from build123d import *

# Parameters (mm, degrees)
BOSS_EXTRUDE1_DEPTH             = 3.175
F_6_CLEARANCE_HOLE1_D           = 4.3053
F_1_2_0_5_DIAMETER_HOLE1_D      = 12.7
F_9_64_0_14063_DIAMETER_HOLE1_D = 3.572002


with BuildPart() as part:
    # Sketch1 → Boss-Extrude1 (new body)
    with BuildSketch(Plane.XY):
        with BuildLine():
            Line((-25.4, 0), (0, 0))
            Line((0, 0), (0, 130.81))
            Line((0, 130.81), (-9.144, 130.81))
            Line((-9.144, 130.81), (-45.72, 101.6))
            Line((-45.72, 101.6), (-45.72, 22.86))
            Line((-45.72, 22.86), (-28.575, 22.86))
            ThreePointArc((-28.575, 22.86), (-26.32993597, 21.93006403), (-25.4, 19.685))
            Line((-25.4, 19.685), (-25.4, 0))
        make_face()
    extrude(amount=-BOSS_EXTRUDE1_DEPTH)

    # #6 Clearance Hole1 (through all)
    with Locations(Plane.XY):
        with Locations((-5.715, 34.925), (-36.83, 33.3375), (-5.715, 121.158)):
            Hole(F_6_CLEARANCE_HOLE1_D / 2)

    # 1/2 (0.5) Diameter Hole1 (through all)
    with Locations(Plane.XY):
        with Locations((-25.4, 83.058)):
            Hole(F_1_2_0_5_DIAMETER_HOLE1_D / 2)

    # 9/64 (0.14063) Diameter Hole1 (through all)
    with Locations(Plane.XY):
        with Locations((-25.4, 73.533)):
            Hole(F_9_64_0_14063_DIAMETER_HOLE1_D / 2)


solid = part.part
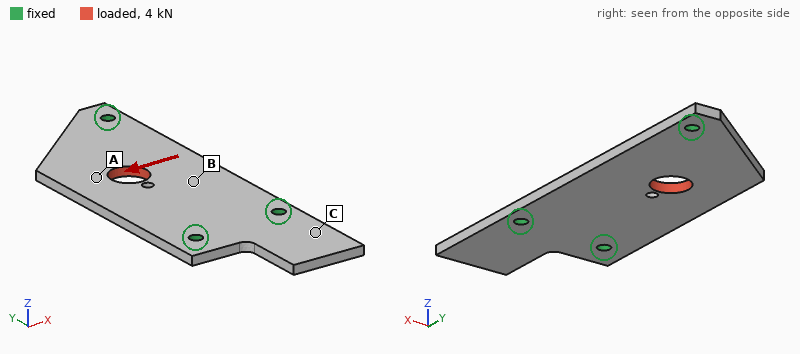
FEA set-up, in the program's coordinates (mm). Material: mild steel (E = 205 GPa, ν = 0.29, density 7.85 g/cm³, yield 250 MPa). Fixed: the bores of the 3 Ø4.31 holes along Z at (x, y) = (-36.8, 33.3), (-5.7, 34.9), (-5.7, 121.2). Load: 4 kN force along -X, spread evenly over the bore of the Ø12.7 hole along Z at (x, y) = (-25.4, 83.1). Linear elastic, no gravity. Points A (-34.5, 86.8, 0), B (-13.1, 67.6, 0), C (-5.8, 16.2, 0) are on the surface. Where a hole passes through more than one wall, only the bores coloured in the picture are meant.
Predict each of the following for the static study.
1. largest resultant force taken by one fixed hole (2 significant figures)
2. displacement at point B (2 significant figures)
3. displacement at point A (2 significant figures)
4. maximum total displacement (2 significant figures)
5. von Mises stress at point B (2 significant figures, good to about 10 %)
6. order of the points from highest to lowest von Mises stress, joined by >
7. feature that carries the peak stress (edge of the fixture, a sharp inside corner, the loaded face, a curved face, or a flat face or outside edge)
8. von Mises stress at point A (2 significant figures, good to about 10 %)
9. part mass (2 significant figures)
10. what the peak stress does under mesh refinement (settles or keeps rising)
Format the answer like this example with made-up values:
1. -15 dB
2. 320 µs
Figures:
1. 2.2 kN
2. 11 µm
3. 14 µm
4. 15 µm
5. 30 MPa
6. A > B > C
7. edge of the fixture
8. 43 MPa
9. 120 g
10. keeps rising
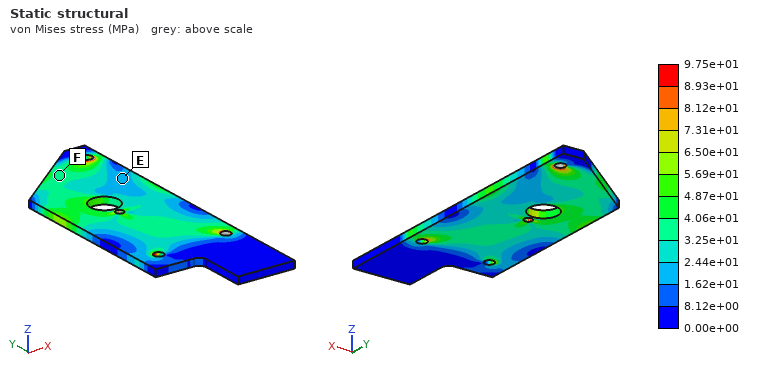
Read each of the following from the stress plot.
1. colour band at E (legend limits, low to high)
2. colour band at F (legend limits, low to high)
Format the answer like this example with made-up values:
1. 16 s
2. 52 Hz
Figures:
1. 1.62e+01 to 2.44e+01 MPa
2. 3.25e+01 to 4.06e+01 MPa
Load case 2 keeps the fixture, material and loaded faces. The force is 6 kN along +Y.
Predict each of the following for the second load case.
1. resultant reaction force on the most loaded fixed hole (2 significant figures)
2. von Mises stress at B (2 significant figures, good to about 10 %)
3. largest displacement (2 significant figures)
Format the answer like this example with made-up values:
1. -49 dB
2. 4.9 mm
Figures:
1. 2.2 kN
2. 31 MPa
3. 11 µm
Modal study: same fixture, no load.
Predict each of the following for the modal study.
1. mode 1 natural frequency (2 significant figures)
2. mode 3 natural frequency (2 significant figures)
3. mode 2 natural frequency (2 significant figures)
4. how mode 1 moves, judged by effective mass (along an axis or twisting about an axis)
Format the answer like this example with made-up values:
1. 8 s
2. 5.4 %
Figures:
1. 1600 Hz
2. 2800 Hz
3. 2300 Hz
4. along Z
